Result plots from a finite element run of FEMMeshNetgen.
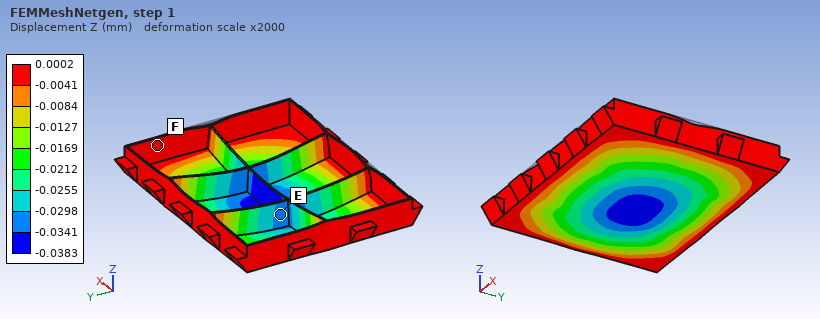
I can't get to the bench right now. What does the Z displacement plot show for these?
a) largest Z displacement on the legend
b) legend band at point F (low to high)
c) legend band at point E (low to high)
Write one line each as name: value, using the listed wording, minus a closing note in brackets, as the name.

largest Z displacement on the legend: 0.0002 mm
legend band at point F: -0.0041 to 0.0002 mm
legend band at point E: -0.0341 to -0.0298 mm
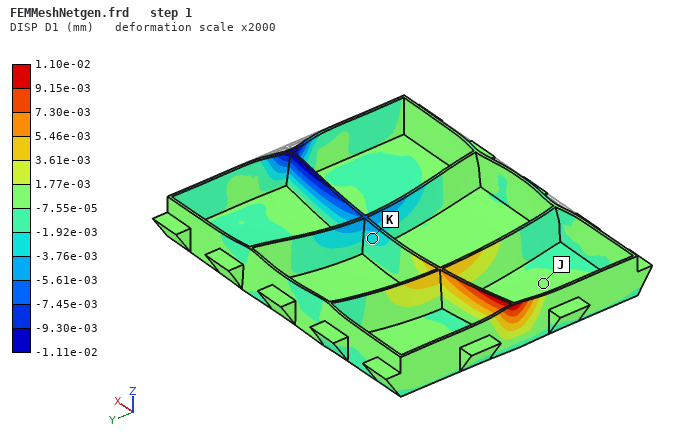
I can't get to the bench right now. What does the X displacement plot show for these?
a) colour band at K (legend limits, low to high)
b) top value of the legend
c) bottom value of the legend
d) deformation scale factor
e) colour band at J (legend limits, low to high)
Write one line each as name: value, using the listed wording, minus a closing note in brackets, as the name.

colour band at K: -3.76e-03 to -1.92e-03 mm
top value of the legend: 1.10e-02 mm
bottom value of the legend: -1.11e-02 mm
deformation scale factor: 2000
colour band at J: -7.55e-05 to 1.77e-03 mm
